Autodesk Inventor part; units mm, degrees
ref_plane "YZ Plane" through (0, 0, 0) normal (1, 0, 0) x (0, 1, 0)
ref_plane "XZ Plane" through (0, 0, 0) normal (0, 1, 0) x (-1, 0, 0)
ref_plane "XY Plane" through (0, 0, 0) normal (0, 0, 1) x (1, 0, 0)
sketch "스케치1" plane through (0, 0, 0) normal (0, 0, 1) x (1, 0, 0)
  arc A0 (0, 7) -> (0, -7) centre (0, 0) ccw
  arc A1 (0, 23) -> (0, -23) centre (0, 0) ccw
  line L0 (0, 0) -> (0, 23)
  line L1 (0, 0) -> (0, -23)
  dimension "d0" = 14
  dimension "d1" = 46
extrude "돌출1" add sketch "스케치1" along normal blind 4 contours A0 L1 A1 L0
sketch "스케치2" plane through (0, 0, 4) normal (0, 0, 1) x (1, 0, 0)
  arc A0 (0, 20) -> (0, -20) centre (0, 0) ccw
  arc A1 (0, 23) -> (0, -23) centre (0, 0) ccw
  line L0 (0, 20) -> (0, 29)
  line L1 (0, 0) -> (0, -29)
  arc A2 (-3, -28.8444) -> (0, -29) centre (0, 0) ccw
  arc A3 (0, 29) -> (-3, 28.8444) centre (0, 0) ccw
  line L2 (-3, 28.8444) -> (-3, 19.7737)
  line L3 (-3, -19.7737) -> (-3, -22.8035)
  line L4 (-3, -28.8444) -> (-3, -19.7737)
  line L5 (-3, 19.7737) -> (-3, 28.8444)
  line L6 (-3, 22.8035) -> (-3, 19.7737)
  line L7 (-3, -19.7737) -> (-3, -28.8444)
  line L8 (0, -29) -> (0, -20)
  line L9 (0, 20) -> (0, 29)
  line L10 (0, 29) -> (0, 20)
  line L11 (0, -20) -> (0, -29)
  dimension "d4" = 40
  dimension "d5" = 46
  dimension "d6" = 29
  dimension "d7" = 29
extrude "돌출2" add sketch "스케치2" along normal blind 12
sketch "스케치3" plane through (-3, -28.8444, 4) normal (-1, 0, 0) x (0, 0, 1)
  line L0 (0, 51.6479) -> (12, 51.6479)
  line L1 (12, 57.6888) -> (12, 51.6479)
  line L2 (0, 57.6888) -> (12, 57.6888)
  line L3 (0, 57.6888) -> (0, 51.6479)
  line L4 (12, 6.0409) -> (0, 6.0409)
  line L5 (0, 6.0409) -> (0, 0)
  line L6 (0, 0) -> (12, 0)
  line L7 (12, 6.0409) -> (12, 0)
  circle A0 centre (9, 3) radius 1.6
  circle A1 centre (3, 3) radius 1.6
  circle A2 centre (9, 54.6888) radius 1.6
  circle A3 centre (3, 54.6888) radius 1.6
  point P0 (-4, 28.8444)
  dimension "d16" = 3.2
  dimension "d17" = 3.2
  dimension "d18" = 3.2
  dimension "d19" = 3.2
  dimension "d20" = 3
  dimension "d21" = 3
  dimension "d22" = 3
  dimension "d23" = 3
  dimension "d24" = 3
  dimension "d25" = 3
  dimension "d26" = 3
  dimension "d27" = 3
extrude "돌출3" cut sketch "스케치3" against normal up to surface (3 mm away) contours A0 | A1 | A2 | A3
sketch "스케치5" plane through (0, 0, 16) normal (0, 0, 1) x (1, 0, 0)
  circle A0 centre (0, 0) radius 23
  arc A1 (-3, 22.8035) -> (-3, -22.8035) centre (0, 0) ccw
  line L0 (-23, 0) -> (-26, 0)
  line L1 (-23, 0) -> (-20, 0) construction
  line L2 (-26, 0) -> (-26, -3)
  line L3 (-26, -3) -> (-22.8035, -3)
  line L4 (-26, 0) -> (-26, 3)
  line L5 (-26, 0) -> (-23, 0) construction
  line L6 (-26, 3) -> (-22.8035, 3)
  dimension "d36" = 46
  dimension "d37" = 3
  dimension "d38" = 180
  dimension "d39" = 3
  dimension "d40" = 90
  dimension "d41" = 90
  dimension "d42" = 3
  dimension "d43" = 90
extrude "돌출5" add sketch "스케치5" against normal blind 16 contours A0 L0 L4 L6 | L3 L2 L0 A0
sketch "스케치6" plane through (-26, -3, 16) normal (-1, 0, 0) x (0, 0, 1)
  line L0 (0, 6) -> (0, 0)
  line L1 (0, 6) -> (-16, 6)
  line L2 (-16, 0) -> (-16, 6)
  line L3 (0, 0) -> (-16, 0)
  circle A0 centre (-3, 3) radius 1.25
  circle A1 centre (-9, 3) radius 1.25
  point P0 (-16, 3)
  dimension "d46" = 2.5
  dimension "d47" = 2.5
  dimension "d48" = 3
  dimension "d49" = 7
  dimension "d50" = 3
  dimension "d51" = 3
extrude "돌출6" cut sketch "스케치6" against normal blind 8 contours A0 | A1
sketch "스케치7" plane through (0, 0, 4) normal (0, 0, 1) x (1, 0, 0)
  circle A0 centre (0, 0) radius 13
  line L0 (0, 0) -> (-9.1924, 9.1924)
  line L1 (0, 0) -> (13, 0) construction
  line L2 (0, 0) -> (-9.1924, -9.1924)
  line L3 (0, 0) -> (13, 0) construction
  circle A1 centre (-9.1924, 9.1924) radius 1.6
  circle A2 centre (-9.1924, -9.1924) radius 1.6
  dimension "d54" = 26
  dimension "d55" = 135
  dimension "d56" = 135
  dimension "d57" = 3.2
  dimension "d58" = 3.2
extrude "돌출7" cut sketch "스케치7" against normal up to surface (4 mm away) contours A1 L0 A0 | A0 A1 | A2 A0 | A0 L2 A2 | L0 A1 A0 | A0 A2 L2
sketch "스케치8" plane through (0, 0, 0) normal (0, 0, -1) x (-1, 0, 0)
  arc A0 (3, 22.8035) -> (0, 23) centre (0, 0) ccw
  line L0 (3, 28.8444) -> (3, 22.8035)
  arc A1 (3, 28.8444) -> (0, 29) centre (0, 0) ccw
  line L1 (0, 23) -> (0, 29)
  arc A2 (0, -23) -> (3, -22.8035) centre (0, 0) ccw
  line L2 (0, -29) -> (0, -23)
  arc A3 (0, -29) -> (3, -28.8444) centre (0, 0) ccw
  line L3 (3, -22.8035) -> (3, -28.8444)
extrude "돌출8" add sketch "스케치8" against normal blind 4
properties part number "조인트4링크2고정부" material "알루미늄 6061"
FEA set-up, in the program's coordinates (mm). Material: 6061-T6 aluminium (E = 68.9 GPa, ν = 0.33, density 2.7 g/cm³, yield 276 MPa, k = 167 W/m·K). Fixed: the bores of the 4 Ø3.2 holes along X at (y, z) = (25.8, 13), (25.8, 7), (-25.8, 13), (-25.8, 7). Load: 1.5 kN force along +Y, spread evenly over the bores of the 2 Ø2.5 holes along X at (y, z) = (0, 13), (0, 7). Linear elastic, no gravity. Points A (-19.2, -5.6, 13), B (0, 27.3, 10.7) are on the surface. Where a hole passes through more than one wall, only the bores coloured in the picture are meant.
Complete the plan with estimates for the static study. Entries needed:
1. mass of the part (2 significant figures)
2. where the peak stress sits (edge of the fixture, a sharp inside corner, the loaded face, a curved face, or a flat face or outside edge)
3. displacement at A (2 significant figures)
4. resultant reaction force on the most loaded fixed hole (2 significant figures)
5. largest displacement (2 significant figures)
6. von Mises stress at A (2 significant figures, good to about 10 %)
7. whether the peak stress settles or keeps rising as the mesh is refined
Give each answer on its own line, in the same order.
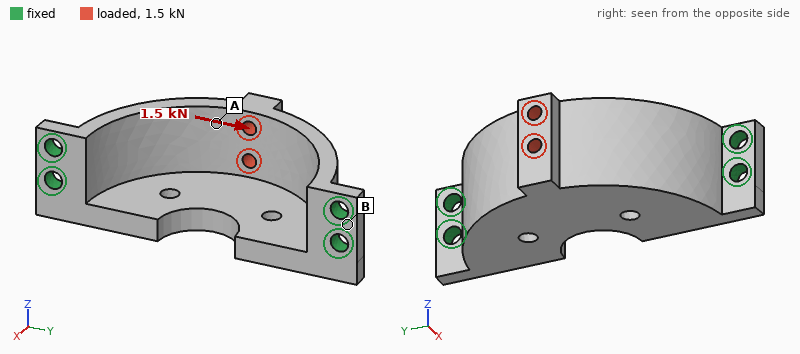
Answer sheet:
16 g
edge of the fixture
42 µm
1.0 kN
57 µm
47 MPa
keeps rising
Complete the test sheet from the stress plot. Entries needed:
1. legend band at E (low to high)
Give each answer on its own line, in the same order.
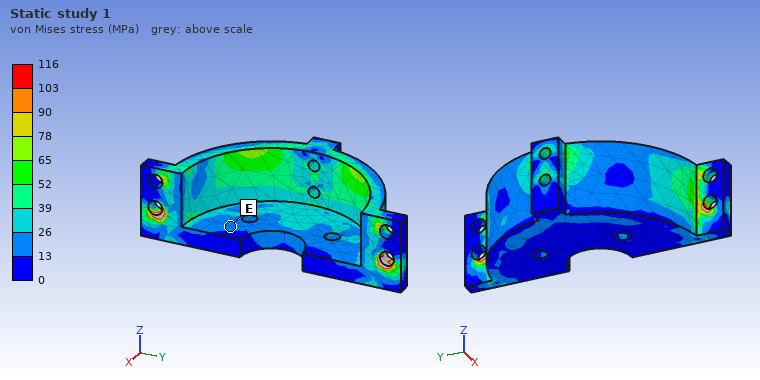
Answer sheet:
13 to 26 MPa
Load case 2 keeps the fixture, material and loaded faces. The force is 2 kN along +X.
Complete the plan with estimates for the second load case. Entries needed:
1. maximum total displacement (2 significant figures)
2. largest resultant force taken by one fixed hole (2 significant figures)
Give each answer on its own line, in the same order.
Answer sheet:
0.10 mm
650 N
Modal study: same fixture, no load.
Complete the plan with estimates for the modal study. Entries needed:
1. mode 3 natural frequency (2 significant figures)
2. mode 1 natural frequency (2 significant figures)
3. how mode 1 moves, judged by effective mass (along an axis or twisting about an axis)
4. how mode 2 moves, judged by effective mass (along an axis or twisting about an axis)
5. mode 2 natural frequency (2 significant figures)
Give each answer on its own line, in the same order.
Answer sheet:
15 kHz
5700 Hz
along Z
along Y
11 kHz
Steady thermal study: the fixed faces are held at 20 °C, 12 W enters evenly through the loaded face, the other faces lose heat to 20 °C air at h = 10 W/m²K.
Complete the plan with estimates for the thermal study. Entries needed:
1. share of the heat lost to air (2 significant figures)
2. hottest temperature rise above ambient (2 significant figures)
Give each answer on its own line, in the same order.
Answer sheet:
3.1 %
21 K
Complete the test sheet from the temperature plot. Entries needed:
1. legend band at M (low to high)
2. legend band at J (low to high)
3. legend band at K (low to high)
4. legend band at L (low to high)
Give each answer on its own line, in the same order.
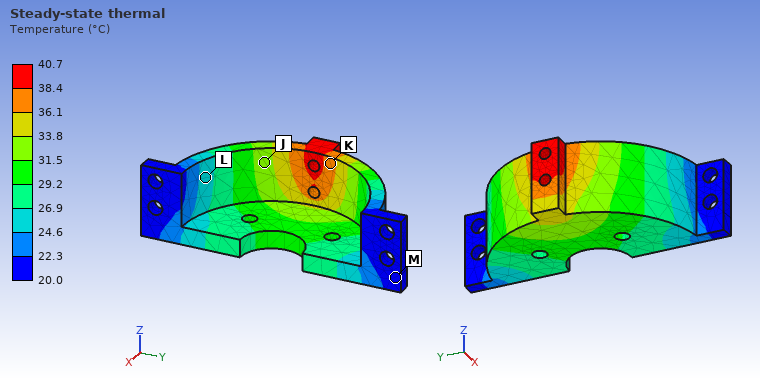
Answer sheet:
20.0 to 22.3 °C
31.5 to 33.8 °C
36.1 to 38.4 °C
24.6 to 26.9 °C
